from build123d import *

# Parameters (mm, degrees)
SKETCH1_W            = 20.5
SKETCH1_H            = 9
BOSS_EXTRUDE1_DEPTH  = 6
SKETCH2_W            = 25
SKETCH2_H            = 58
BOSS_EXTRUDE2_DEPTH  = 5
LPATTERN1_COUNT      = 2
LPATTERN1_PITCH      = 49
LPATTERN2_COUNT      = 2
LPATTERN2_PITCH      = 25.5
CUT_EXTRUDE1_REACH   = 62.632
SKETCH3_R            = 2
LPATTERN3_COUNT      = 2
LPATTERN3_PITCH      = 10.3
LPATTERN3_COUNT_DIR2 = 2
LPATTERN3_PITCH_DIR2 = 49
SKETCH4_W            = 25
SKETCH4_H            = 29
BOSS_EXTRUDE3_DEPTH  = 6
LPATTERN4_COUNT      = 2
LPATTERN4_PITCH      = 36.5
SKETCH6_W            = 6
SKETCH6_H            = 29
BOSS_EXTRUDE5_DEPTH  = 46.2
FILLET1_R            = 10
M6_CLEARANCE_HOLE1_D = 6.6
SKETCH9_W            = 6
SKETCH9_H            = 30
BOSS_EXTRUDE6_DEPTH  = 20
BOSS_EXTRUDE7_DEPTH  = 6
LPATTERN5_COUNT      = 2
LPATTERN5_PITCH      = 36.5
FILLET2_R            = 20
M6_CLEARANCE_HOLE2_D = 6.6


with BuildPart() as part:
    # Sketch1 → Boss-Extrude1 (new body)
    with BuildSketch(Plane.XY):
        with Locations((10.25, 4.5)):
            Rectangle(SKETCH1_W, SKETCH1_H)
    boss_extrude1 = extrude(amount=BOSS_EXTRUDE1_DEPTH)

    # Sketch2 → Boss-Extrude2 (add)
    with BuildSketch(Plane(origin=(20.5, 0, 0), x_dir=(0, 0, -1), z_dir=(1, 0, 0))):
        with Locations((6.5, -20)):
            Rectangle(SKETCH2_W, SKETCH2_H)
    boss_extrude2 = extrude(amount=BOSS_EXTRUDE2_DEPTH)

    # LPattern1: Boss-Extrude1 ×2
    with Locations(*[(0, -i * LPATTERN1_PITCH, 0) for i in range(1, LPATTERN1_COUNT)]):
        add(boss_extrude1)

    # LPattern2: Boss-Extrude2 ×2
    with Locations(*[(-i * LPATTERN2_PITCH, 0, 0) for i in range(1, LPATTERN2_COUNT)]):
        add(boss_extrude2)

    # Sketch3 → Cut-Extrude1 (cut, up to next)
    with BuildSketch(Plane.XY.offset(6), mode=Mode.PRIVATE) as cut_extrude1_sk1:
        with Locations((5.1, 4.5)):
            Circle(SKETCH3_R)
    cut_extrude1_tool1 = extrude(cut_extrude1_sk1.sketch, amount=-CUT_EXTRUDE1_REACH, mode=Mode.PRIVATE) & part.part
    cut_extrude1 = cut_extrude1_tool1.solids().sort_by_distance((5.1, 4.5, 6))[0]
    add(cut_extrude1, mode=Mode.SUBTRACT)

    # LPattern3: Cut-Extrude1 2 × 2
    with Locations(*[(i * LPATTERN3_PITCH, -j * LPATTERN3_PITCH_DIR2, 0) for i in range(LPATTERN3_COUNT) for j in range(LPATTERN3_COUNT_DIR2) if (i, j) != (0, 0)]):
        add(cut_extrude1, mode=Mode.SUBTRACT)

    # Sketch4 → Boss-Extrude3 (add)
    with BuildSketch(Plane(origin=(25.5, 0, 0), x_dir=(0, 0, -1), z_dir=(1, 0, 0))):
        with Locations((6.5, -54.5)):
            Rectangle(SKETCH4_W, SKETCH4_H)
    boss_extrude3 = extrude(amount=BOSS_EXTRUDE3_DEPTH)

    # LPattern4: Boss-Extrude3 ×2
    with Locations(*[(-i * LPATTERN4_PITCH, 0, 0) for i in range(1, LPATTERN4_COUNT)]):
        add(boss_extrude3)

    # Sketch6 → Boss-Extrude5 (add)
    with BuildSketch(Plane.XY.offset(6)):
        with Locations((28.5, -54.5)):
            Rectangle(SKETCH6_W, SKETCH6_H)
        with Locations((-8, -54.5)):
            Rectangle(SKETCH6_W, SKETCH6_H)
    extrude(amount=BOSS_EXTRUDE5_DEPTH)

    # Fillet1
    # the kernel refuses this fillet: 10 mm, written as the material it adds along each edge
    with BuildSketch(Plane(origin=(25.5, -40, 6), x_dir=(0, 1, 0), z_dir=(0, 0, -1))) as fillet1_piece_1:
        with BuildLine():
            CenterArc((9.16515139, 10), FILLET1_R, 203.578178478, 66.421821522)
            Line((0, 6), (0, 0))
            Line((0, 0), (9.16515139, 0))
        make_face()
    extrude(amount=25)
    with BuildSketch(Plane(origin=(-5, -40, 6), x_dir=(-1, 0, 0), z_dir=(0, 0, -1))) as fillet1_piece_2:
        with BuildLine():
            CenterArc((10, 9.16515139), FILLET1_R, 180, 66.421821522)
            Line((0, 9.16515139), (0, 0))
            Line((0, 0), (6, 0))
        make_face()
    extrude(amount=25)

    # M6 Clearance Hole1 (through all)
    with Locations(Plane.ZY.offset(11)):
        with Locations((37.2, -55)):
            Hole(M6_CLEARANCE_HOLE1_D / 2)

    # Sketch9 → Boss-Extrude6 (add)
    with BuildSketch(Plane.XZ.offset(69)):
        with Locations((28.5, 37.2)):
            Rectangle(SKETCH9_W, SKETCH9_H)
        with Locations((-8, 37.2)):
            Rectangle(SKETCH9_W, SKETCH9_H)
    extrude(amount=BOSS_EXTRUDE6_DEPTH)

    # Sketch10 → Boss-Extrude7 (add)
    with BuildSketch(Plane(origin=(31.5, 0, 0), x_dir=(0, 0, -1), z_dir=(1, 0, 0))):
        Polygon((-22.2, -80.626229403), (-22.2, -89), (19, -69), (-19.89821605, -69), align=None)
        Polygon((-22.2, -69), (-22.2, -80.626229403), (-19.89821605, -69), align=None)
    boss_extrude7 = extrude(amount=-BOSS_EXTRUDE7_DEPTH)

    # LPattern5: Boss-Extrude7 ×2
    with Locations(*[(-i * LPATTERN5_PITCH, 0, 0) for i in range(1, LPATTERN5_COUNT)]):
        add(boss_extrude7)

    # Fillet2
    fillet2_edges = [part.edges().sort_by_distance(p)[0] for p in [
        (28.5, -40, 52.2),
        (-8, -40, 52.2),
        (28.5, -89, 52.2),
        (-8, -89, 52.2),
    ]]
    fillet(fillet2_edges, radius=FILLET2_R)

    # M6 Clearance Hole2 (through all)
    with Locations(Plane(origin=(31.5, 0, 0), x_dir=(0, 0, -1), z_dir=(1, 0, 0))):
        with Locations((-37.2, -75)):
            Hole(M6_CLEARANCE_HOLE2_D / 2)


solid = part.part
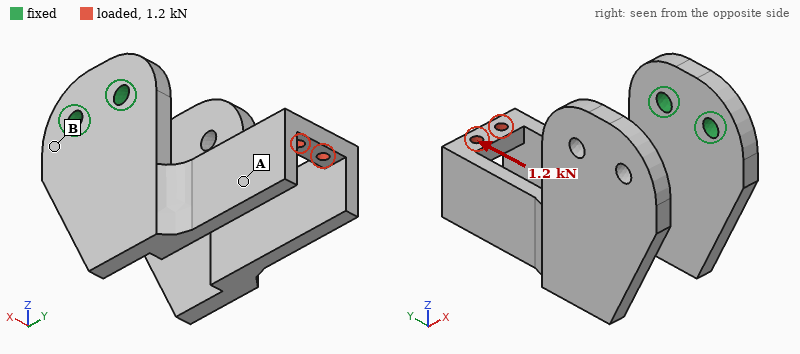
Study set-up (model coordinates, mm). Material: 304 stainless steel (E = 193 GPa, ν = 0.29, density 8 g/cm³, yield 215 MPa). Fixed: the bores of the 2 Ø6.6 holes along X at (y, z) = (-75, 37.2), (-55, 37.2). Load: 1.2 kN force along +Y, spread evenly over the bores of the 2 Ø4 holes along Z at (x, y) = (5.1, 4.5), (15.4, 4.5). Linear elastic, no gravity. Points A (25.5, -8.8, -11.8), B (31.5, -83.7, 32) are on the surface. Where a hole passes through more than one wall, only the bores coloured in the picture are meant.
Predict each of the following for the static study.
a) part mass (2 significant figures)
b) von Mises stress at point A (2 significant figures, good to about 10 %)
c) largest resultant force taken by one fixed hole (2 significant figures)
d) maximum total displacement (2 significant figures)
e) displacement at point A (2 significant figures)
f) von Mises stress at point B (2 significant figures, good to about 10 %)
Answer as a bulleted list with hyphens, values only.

- 410 g
- 18 MPa
- 1.8 kN
- 0.39 mm
- 0.23 mm
- 41 MPa
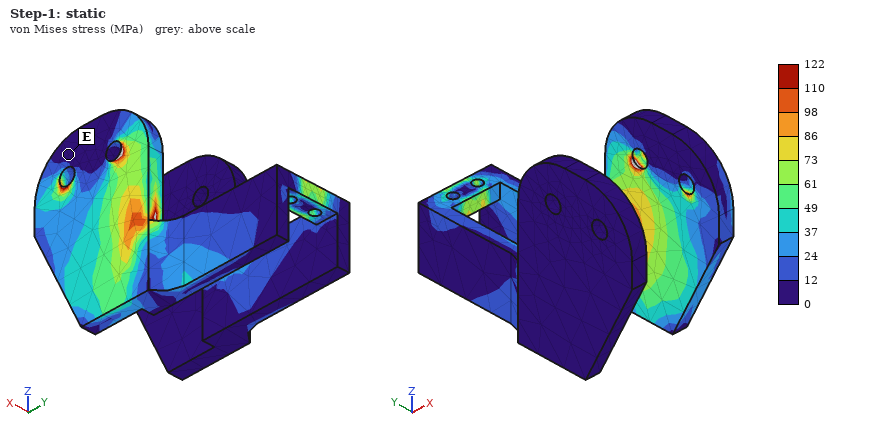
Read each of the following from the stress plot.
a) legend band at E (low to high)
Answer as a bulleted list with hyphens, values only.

- 0 to 12 MPa
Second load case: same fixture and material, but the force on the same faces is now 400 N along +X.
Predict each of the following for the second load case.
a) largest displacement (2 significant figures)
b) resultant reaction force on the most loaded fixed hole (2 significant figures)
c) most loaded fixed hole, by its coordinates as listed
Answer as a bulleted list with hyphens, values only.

- 0.50 mm
- 1.1 kN
- (-55, 37.2)
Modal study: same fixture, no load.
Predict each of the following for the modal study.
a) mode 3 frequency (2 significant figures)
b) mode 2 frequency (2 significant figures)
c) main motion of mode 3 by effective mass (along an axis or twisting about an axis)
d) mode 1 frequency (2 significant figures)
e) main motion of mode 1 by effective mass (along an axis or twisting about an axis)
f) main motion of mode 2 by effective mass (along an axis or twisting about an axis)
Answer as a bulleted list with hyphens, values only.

- 760 Hz
- 480 Hz
- along X
- 340 Hz
- along Z
- along Y
